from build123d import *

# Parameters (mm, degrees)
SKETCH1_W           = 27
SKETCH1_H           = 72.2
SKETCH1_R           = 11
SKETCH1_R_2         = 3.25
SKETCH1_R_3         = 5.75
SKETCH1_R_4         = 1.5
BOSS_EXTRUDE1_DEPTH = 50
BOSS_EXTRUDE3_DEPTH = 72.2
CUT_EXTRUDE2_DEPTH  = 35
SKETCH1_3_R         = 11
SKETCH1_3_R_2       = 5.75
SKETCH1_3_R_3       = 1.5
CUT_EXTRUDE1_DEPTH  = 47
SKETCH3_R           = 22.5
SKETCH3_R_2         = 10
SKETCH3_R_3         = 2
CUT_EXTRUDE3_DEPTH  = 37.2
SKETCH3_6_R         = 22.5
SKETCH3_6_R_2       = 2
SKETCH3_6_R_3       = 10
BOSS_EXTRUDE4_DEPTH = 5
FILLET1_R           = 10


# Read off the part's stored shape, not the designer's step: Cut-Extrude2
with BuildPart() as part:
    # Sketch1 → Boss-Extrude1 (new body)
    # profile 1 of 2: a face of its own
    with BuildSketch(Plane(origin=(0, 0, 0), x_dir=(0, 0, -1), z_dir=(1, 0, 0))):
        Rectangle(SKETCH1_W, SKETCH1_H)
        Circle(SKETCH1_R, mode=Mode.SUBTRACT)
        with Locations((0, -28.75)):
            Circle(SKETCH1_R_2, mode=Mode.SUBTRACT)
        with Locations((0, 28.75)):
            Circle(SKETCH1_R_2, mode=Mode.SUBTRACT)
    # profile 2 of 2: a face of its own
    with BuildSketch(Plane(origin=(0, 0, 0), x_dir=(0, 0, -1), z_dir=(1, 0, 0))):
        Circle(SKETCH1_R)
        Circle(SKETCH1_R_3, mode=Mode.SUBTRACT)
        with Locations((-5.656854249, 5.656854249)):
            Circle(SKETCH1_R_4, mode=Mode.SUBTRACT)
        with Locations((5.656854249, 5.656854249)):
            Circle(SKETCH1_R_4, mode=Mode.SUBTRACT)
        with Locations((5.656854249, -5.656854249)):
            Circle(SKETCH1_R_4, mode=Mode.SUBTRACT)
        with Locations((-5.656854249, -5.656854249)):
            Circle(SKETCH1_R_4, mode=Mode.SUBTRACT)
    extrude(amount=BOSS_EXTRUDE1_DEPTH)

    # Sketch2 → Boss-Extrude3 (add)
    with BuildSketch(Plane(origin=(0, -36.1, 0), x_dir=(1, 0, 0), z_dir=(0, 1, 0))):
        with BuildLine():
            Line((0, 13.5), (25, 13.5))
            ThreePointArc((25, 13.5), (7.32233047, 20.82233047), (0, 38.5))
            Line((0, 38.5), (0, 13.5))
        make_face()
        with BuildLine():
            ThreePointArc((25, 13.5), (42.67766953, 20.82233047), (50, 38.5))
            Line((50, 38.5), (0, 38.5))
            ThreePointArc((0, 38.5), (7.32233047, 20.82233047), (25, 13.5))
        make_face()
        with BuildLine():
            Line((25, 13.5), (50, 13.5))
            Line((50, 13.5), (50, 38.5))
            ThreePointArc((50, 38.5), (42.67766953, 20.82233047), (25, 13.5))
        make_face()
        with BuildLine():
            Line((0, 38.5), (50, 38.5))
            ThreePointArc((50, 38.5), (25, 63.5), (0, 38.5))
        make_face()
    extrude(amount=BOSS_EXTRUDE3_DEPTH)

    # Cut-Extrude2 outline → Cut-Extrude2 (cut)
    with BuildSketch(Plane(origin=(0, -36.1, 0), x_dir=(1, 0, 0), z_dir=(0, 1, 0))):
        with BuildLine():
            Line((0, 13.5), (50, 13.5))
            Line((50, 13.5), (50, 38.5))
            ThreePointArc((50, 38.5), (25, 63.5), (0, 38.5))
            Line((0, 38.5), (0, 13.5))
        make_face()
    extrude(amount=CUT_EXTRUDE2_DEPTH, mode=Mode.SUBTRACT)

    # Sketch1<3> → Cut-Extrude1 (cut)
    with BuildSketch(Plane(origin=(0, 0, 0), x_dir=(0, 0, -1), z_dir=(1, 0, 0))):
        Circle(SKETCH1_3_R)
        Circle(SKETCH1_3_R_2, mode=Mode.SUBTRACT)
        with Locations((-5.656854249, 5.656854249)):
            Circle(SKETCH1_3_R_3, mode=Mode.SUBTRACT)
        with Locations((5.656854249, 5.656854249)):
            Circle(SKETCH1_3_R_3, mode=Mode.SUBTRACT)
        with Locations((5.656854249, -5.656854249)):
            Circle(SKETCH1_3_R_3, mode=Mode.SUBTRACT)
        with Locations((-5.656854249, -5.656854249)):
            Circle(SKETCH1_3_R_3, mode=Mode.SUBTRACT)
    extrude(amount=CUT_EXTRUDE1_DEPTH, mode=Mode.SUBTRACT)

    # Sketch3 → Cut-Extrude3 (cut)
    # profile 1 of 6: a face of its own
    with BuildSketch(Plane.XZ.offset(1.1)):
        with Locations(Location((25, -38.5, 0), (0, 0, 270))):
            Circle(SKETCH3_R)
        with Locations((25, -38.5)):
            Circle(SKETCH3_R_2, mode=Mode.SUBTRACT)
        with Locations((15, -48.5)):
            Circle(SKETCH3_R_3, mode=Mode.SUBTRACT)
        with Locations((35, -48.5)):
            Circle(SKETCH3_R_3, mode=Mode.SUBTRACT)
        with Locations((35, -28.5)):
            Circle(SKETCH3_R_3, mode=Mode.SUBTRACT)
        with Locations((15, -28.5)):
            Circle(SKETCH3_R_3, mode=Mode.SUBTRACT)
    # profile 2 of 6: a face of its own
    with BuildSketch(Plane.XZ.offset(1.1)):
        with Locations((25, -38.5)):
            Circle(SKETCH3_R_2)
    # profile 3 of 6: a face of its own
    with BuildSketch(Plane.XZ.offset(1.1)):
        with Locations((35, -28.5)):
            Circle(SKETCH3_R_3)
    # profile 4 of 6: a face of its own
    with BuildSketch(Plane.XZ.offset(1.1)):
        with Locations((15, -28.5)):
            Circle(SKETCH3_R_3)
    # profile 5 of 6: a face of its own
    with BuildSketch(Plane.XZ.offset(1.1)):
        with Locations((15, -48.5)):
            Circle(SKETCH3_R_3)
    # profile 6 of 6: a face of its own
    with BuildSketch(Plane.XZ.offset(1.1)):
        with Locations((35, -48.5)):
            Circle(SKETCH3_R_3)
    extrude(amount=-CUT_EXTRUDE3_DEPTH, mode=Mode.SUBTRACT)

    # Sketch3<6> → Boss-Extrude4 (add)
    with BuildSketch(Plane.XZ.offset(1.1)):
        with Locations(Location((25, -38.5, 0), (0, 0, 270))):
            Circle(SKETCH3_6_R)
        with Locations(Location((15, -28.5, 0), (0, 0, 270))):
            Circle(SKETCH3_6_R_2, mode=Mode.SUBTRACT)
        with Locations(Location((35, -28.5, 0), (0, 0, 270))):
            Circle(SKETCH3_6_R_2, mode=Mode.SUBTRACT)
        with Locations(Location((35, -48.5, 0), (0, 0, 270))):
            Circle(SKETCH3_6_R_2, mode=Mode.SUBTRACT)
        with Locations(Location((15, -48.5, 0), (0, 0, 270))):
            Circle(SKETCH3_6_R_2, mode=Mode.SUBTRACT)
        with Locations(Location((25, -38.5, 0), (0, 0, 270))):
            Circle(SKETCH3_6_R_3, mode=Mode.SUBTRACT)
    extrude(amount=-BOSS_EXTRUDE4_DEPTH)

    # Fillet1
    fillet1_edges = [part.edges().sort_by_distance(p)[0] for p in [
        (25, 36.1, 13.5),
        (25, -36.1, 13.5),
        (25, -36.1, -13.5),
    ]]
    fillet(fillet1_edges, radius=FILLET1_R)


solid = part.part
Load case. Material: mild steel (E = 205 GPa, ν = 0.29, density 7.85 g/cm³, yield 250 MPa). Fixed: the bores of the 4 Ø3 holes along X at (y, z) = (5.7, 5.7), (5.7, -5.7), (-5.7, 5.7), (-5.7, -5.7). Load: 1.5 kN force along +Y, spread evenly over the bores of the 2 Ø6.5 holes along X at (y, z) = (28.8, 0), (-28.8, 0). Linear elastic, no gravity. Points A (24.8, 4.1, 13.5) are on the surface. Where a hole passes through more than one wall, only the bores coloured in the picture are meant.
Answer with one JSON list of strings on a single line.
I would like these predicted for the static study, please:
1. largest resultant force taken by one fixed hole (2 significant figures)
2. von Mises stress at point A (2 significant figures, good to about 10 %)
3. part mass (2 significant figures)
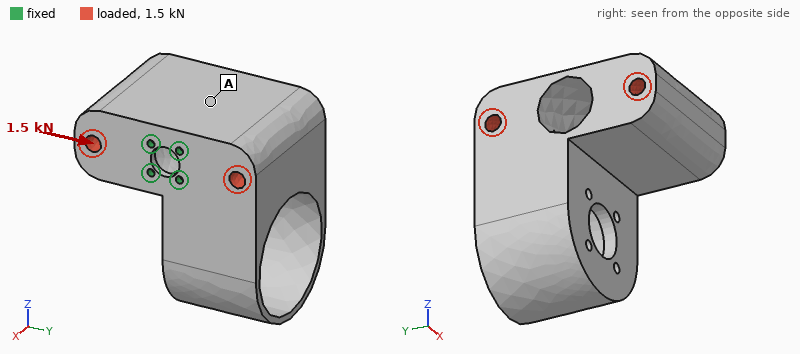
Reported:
["1.2 kN", "11 MPa", "810 g"]
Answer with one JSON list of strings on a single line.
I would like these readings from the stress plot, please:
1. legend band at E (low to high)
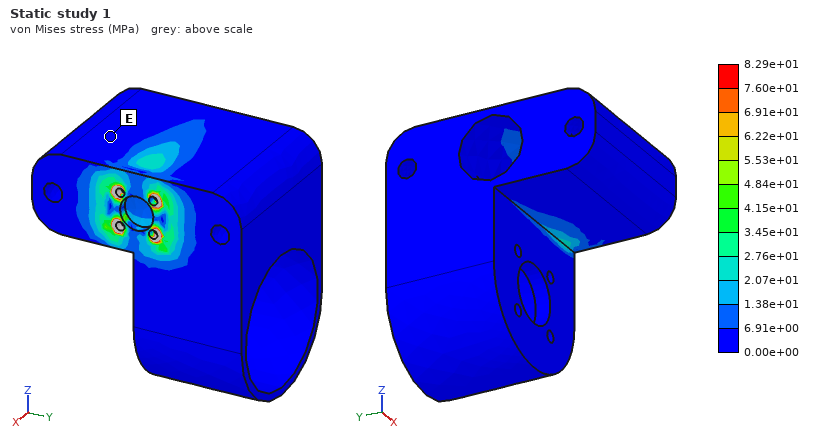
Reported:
["0.00e+00 to 6.91e+00 MPa"]
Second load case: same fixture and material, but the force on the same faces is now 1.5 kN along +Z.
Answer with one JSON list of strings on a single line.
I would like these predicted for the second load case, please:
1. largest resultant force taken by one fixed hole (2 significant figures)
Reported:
["1.2 kN"]
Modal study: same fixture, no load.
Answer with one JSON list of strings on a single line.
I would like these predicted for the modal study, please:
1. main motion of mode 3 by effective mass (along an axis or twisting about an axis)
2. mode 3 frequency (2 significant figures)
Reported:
["twisting about X", "2900 Hz"]
